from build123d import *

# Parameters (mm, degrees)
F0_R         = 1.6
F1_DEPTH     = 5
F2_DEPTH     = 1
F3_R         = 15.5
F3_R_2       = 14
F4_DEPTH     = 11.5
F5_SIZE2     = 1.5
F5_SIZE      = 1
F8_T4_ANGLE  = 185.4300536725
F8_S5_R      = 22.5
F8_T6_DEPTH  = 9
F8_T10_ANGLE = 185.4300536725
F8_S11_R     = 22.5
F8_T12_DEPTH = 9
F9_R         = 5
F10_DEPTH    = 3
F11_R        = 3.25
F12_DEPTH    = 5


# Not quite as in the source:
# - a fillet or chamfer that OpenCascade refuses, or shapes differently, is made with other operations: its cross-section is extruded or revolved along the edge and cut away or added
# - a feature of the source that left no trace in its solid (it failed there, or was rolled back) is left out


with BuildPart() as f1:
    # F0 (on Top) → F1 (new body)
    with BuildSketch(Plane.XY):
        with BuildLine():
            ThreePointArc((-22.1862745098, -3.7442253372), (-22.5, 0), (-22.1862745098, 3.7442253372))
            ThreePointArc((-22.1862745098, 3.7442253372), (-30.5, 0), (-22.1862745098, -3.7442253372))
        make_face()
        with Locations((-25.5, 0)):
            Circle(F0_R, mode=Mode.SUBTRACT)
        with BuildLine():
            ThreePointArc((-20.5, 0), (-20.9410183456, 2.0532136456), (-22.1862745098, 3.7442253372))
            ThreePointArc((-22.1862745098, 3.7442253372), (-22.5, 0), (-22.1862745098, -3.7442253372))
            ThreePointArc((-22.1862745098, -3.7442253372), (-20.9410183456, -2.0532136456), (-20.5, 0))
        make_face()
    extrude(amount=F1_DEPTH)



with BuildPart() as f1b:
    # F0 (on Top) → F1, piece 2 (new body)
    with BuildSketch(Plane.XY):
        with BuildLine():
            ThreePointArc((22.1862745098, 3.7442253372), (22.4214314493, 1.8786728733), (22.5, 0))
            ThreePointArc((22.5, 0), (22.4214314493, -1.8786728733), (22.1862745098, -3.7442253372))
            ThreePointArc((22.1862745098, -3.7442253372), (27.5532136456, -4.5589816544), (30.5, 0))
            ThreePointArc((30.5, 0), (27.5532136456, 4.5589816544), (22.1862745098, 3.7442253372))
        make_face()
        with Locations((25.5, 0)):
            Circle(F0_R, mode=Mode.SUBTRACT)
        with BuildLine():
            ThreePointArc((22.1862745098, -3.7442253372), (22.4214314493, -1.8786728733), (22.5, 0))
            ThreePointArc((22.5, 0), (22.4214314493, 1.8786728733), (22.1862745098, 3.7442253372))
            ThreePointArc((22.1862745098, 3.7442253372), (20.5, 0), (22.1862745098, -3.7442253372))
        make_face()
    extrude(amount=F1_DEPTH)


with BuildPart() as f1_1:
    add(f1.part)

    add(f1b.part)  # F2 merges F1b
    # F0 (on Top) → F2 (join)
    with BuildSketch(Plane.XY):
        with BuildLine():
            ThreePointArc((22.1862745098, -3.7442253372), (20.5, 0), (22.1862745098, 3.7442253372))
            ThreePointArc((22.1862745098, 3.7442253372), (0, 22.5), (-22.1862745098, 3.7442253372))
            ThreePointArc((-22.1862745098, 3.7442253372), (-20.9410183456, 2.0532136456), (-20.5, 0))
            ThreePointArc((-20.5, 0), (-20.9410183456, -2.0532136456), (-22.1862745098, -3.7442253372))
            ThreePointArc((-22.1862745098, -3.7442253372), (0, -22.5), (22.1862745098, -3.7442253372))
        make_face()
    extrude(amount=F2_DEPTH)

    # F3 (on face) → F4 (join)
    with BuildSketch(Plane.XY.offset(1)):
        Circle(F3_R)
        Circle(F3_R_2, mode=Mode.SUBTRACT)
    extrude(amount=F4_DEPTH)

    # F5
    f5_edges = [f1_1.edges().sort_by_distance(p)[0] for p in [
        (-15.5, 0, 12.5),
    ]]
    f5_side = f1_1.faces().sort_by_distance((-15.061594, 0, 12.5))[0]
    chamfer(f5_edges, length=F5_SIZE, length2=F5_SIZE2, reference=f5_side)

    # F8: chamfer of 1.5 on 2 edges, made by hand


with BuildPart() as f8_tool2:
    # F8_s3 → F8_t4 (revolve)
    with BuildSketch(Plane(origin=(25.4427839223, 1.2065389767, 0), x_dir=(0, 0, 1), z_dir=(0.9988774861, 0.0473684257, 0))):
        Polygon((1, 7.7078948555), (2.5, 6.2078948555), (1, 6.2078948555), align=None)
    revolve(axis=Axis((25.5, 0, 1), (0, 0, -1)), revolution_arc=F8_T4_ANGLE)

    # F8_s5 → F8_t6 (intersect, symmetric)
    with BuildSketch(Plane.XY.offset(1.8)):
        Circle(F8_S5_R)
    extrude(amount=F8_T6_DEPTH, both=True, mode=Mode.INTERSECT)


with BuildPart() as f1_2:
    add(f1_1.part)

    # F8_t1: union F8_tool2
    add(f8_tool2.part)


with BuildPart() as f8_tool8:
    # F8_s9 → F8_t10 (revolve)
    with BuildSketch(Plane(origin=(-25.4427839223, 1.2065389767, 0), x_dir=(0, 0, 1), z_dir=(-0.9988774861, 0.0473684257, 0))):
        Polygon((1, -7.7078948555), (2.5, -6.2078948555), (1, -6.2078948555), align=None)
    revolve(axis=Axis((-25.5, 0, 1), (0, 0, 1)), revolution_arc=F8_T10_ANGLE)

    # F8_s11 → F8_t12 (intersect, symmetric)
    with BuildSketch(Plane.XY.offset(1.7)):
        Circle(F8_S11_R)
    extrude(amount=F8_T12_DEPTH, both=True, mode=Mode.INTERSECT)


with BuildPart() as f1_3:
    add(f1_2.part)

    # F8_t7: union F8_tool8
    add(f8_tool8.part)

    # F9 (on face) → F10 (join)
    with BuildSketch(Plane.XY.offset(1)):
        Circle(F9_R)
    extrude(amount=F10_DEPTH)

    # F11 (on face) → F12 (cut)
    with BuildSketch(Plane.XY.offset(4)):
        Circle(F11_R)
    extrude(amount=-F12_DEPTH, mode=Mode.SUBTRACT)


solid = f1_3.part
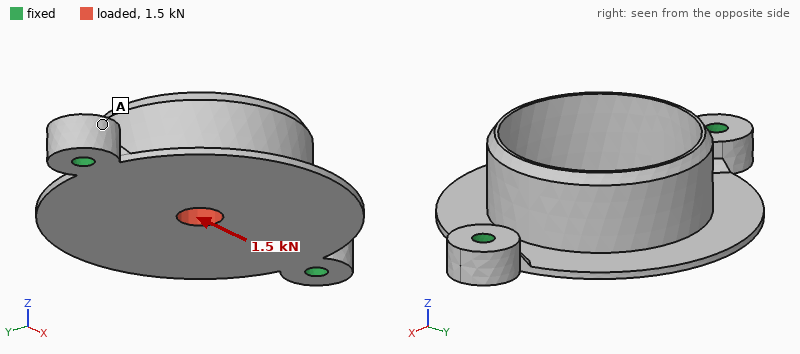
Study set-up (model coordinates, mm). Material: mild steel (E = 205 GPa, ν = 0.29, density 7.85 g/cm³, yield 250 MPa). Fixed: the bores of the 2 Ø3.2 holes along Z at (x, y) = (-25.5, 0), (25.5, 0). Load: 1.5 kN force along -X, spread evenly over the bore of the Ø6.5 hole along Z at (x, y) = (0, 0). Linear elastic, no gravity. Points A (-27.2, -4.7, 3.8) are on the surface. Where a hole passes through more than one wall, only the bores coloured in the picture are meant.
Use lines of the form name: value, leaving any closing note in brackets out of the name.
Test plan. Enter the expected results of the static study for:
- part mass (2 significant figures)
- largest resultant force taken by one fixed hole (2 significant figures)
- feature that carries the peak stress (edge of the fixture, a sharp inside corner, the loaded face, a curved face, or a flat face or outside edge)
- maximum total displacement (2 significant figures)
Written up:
part mass: 31 g
largest resultant force taken by one fixed hole: 750 N
feature that carries the peak stress: a flat face or outside edge
maximum total displacement: 29 µm
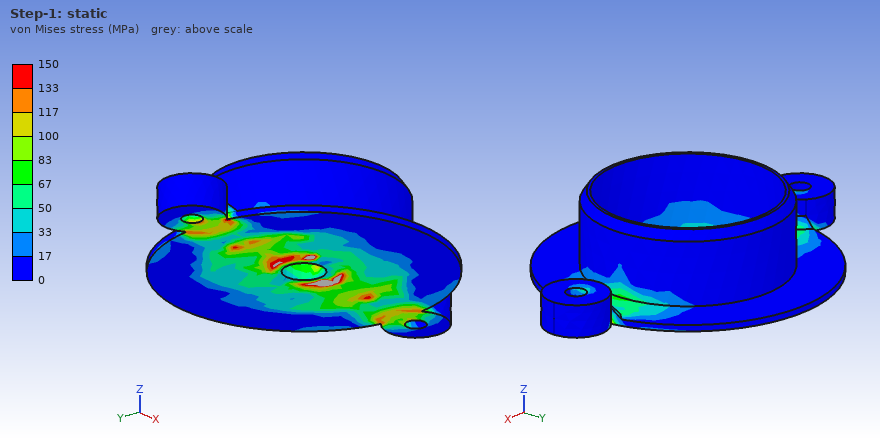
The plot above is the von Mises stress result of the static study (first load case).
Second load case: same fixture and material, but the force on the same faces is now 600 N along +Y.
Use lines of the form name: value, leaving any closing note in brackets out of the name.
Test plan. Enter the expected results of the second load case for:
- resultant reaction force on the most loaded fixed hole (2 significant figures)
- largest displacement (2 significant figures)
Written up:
resultant reaction force on the most loaded fixed hole: 300 N
largest displacement: 50 µm
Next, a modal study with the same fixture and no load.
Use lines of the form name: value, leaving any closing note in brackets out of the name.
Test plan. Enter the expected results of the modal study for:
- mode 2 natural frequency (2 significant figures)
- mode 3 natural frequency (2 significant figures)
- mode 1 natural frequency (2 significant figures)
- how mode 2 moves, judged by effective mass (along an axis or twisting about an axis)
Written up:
mode 2 natural frequency: 3200 Hz
mode 3 natural frequency: 6700 Hz
mode 1 natural frequency: 1600 Hz
how mode 2 moves, judged by effective mass: along Z
